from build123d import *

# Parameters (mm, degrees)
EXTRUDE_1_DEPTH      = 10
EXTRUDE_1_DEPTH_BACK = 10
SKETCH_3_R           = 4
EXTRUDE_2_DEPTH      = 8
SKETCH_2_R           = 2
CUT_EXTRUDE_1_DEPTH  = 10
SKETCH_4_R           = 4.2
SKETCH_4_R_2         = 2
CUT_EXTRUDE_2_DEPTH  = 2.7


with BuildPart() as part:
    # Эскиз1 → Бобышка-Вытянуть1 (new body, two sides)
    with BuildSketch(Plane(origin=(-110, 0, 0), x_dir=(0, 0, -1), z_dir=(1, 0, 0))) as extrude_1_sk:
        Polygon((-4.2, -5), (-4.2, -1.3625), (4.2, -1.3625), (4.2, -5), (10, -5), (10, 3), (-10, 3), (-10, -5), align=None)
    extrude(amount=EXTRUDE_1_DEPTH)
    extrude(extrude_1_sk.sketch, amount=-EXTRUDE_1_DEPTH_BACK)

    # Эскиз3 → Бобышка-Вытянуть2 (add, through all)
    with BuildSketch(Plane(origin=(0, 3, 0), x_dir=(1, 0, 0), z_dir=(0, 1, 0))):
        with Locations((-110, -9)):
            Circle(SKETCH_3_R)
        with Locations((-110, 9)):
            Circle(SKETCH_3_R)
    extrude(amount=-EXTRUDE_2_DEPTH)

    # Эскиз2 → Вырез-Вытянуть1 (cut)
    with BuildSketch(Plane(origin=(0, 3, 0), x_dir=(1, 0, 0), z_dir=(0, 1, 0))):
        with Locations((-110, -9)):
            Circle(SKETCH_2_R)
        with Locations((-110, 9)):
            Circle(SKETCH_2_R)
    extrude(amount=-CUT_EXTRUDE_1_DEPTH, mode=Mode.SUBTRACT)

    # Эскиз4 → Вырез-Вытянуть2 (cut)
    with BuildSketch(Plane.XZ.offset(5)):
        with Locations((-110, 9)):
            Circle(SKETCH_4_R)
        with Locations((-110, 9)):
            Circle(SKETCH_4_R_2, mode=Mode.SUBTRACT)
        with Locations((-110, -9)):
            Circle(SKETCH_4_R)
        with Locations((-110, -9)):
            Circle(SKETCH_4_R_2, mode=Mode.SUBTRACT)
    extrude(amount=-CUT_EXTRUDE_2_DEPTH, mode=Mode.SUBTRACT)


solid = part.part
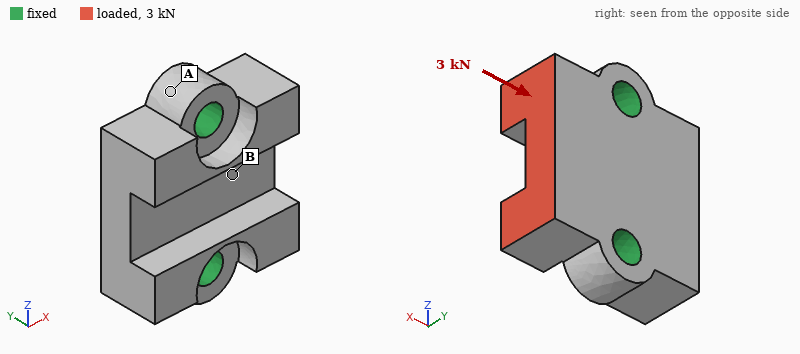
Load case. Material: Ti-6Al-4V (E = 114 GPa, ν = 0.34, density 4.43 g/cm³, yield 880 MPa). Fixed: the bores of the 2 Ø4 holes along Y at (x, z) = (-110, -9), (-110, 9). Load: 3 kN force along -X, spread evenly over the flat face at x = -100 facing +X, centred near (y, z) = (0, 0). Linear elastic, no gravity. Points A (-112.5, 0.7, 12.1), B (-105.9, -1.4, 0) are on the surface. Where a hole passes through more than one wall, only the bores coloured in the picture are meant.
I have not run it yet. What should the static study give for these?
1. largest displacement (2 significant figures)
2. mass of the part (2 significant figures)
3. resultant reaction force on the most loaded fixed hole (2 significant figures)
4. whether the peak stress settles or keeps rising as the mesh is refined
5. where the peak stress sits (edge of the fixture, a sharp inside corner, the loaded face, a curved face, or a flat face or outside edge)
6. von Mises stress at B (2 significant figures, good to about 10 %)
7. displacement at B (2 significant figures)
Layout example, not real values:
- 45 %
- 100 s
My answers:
- 6.1 µm
- 11 g
- 1.5 kN
- keeps rising
- a sharp inside corner
- 21 MPa
- 2.5 µm
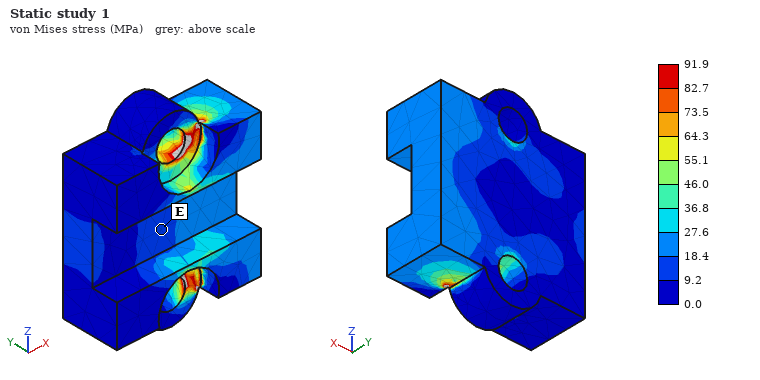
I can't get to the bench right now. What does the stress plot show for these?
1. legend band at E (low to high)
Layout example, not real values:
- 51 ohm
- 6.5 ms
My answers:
- 9.2 to 18.4 MPa
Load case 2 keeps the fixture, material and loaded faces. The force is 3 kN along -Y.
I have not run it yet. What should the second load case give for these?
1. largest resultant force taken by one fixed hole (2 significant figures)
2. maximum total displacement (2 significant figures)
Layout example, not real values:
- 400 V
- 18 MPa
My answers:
- 1.5 kN
- 45 µm
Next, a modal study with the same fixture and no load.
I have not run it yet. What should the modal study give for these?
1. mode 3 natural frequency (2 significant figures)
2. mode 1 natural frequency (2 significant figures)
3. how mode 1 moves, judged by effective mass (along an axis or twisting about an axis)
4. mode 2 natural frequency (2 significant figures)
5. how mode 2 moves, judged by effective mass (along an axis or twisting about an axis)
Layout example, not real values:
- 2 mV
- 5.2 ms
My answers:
- 45 kHz
- 30 kHz
- twisting about Z
- 37 kHz
- along Y
